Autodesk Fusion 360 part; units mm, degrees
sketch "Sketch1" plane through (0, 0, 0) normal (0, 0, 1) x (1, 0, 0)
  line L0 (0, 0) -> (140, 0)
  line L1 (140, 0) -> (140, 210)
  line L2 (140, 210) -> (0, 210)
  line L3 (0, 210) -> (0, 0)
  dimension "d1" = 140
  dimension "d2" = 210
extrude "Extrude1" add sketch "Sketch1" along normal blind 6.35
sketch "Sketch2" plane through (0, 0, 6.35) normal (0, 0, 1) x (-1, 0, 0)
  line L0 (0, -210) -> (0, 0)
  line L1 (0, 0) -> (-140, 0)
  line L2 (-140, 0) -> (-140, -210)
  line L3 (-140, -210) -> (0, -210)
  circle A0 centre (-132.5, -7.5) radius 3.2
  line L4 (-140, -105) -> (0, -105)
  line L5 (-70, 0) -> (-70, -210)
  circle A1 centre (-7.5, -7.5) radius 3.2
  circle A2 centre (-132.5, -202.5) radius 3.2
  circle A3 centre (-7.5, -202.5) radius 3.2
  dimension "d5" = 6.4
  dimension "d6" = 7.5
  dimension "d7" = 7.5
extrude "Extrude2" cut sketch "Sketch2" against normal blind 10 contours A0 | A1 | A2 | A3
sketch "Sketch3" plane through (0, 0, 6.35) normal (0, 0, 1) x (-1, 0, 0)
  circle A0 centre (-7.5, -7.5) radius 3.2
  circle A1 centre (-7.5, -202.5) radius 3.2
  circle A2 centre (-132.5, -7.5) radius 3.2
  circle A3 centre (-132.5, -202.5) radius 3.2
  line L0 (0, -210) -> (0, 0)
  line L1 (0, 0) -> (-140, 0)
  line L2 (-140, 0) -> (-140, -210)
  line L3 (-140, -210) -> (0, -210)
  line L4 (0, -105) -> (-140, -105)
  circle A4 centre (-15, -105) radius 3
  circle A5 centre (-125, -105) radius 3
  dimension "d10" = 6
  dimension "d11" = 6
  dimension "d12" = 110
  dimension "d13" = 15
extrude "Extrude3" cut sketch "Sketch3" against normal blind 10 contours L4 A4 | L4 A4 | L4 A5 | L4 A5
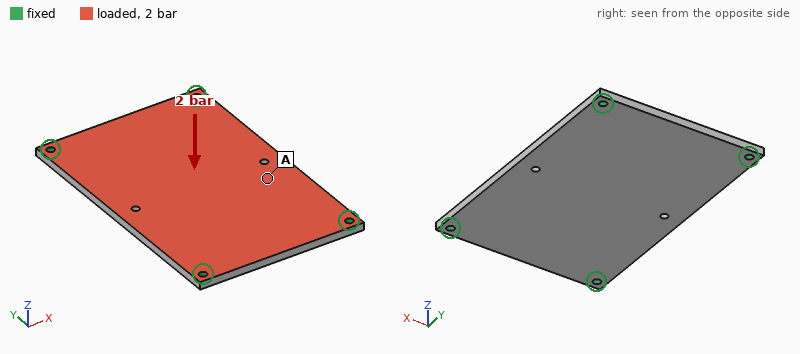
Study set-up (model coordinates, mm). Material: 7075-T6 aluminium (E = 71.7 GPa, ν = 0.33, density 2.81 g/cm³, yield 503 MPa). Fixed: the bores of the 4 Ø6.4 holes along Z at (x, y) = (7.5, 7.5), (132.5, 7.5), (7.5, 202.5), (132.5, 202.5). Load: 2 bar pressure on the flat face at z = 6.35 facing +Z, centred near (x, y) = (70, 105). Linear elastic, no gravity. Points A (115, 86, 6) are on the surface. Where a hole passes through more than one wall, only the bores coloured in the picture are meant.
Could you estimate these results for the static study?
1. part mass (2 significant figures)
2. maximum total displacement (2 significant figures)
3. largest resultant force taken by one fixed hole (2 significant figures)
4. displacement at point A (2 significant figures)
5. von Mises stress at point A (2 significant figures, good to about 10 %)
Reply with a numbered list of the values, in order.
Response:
1. 520 g
2. 0.84 mm
3. 1.5 kN
4. 0.76 mm
5. 54 MPa
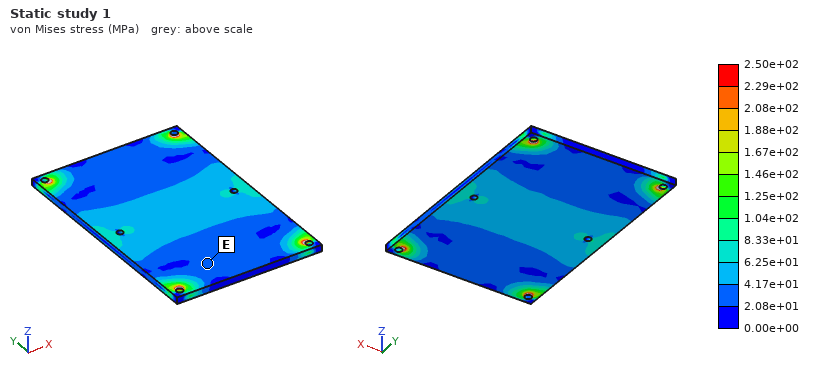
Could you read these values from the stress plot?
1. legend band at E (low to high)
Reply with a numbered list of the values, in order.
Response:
1. 2.08e+01 to 4.17e+01 MPa
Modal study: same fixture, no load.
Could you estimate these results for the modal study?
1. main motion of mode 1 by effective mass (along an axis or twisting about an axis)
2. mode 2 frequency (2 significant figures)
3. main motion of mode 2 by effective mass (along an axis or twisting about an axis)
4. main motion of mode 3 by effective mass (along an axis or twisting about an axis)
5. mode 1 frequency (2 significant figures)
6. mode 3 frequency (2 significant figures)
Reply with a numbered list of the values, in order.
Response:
1. along Z
2. 1100 Hz
3. twisting about Y
4. twisting about X
5. 670 Hz
6. 1700 Hz
